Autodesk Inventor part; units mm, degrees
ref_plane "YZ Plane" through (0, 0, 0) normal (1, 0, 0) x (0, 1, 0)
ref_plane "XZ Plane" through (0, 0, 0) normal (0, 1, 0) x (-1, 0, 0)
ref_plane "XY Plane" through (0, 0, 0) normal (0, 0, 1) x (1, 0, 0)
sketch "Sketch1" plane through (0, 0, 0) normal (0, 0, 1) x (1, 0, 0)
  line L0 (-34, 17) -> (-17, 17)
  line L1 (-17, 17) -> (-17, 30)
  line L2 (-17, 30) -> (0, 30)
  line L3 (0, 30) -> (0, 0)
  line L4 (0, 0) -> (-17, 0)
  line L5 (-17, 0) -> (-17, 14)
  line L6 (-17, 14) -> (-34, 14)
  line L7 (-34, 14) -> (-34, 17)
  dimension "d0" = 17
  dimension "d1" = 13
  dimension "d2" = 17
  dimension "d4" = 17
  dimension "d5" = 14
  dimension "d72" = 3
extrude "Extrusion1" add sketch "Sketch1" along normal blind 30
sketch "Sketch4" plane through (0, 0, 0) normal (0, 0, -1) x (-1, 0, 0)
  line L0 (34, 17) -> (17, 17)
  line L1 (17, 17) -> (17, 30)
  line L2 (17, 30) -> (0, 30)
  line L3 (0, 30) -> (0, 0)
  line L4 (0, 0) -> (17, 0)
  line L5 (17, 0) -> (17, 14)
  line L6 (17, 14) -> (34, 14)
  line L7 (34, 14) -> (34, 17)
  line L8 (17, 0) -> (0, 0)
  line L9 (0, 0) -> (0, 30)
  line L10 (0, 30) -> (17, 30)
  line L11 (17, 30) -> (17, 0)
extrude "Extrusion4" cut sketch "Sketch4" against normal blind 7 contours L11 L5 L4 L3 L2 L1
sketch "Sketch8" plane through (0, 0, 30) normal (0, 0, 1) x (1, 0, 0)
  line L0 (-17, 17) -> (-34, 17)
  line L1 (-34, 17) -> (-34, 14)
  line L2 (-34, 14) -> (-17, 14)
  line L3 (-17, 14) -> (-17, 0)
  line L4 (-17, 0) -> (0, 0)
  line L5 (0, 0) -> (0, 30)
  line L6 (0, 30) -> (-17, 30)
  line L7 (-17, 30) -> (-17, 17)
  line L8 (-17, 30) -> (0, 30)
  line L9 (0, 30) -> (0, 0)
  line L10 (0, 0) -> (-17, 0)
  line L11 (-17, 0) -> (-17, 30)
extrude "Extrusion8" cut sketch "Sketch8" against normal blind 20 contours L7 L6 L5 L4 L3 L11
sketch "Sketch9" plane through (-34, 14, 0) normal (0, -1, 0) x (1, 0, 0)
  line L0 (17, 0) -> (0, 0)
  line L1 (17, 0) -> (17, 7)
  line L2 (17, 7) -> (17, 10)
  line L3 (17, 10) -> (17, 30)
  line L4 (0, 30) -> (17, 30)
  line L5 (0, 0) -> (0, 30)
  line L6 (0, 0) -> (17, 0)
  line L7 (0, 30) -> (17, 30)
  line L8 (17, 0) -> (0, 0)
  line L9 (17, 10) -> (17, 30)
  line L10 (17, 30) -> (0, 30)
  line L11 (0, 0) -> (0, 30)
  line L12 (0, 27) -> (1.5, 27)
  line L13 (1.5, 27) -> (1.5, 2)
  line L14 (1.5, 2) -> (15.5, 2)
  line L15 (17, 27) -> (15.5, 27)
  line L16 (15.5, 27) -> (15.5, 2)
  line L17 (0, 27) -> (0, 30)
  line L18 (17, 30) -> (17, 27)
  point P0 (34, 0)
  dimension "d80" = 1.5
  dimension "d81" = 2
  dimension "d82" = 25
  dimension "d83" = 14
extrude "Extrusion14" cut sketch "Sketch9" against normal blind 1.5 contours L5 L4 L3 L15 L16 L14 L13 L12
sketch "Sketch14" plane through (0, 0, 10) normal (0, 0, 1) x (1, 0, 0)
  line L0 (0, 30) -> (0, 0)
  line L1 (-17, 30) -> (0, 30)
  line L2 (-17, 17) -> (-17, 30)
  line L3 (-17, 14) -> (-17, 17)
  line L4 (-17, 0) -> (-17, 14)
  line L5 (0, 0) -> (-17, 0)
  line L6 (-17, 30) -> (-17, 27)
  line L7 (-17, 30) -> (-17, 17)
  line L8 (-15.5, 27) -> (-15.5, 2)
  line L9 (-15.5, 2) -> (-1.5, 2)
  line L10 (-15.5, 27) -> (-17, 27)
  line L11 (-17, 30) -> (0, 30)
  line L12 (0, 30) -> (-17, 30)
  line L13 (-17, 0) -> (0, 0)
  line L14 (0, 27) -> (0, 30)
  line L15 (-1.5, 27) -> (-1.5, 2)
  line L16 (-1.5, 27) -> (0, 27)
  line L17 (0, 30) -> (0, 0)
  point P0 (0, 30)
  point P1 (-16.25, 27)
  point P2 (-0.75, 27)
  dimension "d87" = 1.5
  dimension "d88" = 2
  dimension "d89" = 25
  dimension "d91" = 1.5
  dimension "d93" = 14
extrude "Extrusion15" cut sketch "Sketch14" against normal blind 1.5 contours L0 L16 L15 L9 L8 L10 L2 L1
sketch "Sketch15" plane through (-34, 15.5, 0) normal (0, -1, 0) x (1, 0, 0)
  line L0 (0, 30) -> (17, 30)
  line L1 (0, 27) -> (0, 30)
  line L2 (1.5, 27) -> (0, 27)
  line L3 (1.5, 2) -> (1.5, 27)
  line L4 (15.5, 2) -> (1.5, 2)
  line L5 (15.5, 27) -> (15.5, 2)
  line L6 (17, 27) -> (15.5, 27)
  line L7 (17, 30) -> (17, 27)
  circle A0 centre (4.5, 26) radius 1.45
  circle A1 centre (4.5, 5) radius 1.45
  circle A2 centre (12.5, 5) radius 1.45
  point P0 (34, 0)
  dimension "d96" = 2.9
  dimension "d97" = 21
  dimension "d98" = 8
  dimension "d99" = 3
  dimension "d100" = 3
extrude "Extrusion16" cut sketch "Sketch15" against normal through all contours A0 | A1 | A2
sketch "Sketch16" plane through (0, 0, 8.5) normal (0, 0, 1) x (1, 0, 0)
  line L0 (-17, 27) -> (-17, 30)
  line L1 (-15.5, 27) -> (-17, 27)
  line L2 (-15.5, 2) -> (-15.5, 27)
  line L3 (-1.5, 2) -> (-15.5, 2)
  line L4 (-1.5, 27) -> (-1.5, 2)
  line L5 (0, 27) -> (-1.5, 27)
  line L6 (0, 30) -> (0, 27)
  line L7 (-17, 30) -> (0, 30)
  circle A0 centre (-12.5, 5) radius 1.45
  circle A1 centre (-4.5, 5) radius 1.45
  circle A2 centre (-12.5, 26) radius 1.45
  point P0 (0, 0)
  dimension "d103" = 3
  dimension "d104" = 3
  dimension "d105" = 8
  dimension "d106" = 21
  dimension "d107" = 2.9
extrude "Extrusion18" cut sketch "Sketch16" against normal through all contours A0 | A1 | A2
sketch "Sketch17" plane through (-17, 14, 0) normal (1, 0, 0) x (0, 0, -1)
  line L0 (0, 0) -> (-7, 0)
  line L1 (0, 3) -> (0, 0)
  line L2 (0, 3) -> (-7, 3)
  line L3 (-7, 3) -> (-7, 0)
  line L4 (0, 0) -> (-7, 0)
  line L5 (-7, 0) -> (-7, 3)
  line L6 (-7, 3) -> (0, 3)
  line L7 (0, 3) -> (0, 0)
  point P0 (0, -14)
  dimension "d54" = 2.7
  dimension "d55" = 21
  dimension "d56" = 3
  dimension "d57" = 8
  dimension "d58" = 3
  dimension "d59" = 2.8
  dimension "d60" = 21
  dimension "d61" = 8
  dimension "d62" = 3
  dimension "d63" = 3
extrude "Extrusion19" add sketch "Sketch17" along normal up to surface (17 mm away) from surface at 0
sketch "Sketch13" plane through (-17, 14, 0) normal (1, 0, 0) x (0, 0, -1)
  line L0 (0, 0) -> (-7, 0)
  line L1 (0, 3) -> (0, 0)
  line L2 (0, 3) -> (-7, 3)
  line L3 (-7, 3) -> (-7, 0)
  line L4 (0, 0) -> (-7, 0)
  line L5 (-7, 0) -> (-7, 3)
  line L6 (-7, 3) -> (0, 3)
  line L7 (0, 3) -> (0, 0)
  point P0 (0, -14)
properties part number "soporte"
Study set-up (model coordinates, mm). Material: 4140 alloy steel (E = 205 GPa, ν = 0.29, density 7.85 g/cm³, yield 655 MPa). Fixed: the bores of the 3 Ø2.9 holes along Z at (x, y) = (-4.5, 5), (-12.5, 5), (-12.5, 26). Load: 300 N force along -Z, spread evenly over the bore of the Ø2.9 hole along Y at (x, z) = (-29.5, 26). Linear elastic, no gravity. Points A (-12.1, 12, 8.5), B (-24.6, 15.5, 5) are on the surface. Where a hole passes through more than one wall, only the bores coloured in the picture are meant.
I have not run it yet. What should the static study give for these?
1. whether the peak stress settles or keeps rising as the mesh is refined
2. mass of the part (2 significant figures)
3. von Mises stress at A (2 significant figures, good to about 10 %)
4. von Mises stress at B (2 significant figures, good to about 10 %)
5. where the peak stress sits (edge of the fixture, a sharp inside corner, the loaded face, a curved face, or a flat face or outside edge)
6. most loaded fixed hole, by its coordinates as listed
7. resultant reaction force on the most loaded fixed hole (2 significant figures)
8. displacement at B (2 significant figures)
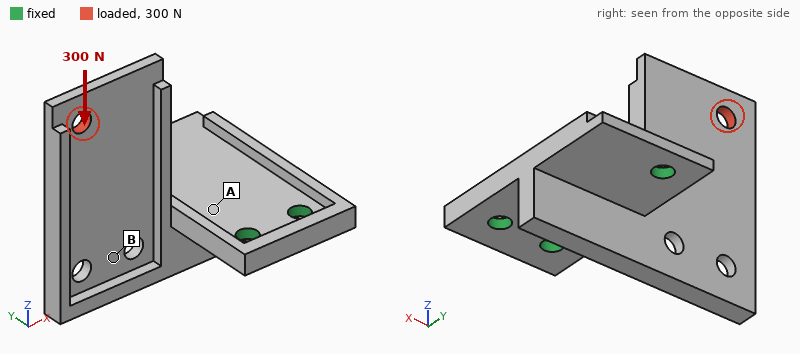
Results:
keeps rising
17 g
150 MPa
74 MPa
edge of the fixture
(-12.5, 5)
380 N
0.091 mm
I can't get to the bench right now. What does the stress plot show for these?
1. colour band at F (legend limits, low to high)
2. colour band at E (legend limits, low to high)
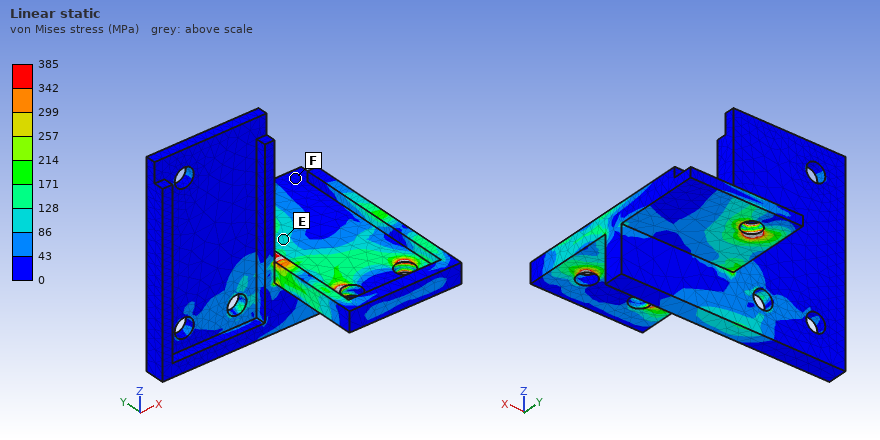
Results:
0 to 43 MPa
86 to 128 MPa
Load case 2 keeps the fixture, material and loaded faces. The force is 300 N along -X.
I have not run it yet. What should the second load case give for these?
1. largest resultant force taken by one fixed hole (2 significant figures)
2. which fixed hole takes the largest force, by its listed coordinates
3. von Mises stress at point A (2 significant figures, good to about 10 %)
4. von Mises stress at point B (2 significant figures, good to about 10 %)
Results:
340 N
(-4.5, 5)
160 MPa
110 MPa
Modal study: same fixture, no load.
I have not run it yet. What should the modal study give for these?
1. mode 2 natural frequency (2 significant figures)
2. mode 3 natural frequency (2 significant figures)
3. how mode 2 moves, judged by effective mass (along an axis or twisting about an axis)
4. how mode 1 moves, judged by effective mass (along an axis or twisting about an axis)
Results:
2800 Hz
4300 Hz
along Z
along Y
